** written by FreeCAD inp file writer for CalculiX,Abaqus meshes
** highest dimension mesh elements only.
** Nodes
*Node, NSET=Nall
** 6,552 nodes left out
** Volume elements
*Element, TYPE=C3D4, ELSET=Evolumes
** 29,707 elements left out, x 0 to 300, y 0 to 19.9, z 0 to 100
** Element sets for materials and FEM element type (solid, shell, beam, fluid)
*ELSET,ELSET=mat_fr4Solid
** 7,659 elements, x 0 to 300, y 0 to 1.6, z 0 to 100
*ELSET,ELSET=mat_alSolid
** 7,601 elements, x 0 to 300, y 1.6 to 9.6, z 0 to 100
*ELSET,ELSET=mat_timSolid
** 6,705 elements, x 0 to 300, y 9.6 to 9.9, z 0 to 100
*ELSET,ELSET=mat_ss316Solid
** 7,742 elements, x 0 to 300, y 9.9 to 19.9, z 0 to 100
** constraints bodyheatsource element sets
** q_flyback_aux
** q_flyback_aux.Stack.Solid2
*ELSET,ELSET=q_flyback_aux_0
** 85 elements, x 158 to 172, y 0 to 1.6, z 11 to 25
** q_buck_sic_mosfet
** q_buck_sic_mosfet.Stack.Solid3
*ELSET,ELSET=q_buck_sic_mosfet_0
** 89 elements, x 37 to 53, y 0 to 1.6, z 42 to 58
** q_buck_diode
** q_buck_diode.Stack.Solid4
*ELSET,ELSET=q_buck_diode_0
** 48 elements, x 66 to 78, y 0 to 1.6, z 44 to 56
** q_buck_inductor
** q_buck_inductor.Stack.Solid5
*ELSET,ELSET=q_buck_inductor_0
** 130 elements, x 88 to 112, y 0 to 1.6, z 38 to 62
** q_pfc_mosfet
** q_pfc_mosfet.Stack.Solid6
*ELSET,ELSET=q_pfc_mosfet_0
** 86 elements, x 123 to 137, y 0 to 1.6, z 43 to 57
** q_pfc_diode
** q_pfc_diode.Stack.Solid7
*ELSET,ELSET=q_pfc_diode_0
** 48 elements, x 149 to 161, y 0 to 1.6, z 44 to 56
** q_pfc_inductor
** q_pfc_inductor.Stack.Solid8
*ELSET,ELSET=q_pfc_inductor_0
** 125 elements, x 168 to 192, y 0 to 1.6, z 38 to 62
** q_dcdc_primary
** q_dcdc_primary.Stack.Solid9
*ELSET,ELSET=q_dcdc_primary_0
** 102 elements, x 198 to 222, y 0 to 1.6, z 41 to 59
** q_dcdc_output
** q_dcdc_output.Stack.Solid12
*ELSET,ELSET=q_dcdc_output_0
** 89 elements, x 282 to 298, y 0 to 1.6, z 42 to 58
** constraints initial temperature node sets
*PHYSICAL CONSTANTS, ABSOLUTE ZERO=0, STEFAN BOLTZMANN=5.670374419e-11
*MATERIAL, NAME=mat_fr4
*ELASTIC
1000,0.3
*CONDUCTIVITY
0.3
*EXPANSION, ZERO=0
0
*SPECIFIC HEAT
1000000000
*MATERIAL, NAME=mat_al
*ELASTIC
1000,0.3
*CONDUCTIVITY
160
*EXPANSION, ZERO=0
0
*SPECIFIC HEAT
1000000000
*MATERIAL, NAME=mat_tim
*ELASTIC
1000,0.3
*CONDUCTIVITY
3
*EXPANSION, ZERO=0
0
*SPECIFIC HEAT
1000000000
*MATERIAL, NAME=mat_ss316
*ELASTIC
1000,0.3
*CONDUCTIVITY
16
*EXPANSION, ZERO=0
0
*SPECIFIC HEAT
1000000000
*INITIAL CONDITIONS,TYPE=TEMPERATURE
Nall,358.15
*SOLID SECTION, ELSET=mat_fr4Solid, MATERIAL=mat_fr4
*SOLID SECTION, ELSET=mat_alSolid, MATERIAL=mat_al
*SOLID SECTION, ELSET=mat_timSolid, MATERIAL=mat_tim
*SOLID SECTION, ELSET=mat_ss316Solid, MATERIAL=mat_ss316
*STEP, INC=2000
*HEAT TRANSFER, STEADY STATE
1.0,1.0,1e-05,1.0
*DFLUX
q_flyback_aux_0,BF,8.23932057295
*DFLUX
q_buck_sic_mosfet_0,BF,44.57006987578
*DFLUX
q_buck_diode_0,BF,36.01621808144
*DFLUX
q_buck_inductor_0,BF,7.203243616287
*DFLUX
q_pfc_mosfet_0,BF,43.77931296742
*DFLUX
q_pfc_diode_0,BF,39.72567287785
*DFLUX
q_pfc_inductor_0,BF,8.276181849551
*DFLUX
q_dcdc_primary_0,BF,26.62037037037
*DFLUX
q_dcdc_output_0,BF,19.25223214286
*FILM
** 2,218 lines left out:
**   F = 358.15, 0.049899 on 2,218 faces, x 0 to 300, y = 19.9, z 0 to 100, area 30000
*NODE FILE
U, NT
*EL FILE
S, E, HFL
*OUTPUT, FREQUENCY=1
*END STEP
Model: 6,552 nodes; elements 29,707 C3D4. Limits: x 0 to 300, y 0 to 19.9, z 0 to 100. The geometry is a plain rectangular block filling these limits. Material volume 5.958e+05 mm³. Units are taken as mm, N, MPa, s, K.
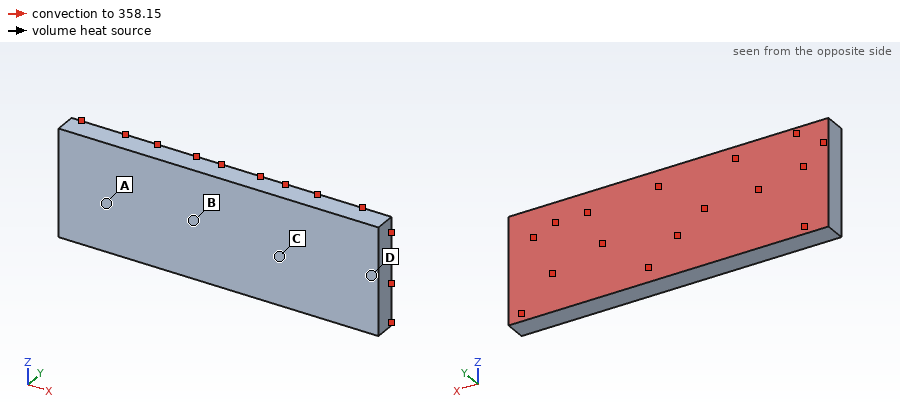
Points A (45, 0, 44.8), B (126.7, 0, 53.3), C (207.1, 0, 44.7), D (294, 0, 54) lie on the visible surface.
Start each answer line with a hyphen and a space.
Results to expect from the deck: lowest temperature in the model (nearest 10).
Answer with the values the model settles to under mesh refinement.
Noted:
- 420 K
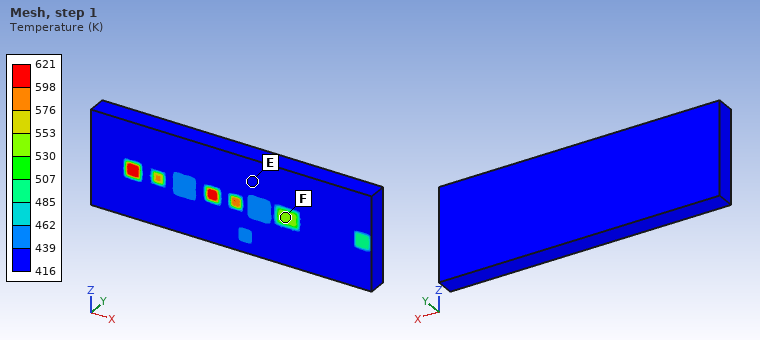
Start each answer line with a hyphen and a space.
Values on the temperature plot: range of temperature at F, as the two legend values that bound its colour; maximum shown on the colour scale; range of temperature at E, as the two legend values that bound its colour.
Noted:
- 530 to 553 K
- 621 K
- 416 to 439 K
